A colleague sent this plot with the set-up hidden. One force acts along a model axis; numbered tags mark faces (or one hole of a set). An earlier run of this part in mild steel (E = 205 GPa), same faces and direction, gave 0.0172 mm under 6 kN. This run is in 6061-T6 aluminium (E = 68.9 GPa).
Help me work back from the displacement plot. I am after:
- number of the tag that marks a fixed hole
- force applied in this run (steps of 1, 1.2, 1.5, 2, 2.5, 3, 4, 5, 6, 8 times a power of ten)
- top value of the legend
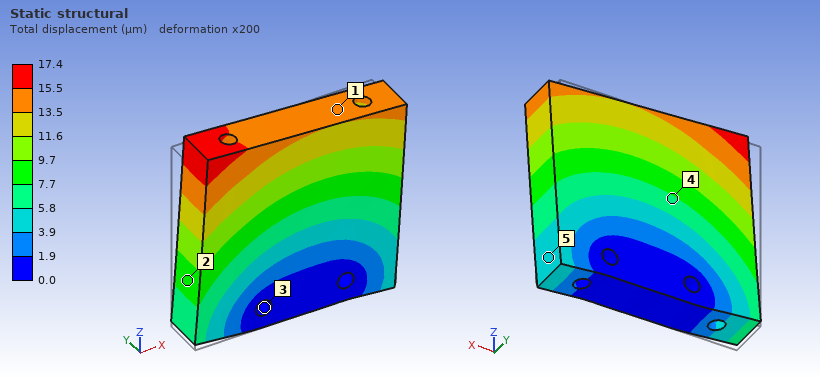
3
2 kN
17.4 µm
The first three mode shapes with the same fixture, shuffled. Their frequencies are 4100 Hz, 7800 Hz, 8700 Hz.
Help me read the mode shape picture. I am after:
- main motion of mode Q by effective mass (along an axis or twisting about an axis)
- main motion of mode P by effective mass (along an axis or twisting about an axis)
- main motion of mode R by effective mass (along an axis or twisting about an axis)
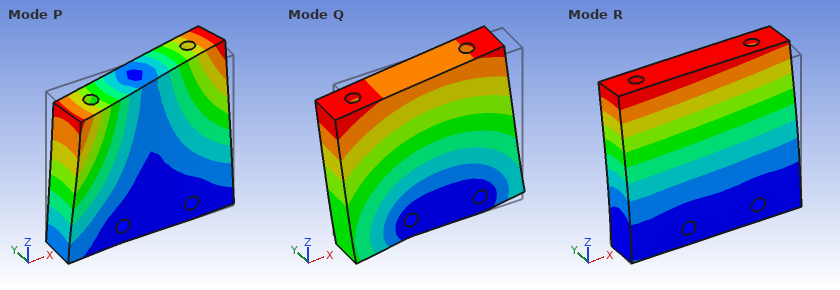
along X
twisting about Z
along Y
